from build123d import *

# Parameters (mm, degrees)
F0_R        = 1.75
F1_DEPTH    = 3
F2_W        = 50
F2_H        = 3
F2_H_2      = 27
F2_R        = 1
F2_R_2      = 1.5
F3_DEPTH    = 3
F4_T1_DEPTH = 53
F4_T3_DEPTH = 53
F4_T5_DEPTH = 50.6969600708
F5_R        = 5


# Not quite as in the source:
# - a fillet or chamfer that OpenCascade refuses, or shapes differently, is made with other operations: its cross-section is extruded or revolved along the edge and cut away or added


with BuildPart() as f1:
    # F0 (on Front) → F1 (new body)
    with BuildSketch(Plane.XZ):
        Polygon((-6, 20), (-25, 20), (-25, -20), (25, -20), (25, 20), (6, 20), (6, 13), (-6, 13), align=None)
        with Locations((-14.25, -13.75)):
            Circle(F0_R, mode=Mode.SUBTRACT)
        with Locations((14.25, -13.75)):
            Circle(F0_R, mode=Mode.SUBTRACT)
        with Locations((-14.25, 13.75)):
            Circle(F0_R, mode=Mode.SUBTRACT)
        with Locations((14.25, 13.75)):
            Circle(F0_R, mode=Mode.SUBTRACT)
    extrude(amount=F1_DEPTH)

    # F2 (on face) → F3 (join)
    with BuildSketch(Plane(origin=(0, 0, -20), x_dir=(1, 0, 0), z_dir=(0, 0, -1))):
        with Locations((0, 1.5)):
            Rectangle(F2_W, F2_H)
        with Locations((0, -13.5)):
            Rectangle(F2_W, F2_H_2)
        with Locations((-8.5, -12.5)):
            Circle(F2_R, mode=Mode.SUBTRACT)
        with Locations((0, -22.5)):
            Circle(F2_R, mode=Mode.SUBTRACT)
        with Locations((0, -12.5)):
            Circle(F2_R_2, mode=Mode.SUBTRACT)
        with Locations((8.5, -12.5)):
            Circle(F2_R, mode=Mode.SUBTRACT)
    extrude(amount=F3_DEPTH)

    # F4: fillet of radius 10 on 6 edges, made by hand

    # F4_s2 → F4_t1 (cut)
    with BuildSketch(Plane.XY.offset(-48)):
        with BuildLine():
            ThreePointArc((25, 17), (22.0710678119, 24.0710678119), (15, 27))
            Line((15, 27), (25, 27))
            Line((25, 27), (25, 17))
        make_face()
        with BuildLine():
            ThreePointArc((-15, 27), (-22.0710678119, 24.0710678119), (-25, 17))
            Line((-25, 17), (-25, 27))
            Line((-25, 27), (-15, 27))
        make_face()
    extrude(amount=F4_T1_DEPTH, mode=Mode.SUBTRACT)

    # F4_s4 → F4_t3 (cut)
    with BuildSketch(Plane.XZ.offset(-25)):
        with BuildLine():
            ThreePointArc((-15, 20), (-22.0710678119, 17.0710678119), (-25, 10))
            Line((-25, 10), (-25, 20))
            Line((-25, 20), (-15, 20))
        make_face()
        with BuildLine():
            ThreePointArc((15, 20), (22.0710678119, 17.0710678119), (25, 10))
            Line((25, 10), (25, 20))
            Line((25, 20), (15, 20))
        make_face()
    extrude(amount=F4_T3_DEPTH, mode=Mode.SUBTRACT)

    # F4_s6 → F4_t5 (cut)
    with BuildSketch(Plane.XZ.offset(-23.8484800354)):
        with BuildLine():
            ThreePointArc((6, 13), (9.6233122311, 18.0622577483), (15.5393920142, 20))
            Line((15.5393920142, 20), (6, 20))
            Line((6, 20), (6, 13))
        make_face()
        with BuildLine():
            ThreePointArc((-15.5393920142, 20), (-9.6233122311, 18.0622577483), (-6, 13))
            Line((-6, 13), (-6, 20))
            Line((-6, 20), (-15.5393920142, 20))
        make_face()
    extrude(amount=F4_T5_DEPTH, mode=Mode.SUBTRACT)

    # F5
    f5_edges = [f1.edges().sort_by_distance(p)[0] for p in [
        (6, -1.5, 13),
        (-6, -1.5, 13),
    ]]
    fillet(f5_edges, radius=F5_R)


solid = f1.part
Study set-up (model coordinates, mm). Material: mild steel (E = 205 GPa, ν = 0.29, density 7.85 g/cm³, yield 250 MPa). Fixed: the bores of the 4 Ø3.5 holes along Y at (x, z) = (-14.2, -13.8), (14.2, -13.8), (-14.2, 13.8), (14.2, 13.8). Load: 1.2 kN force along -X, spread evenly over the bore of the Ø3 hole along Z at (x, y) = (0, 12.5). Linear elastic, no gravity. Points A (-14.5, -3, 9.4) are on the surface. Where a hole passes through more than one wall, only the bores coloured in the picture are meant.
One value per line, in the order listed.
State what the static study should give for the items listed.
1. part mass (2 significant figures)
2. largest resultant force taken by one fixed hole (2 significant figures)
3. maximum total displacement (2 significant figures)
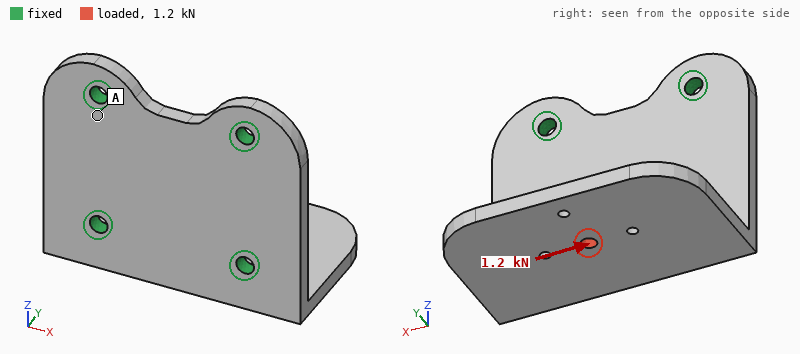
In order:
76 g
850 N
25 µm
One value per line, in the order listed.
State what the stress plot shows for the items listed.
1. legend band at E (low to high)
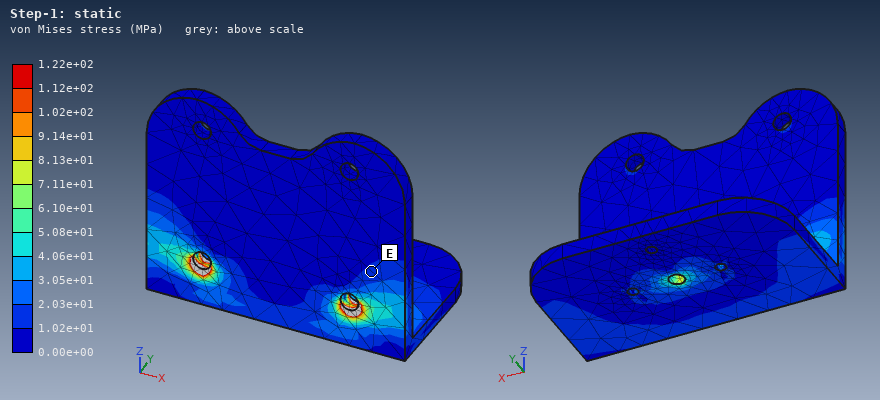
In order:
1.02e+01 to 2.03e+01 MPa
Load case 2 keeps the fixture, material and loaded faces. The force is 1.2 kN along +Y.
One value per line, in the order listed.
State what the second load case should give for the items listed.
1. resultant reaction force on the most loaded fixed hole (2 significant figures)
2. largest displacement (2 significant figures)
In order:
650 N
53 µm
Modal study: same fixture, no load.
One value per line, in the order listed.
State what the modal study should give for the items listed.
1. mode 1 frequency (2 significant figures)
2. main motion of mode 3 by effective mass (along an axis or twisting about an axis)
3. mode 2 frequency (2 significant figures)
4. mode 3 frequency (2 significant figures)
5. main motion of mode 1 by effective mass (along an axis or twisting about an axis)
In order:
2300 Hz
along X
4500 Hz
8100 Hz
along Z
